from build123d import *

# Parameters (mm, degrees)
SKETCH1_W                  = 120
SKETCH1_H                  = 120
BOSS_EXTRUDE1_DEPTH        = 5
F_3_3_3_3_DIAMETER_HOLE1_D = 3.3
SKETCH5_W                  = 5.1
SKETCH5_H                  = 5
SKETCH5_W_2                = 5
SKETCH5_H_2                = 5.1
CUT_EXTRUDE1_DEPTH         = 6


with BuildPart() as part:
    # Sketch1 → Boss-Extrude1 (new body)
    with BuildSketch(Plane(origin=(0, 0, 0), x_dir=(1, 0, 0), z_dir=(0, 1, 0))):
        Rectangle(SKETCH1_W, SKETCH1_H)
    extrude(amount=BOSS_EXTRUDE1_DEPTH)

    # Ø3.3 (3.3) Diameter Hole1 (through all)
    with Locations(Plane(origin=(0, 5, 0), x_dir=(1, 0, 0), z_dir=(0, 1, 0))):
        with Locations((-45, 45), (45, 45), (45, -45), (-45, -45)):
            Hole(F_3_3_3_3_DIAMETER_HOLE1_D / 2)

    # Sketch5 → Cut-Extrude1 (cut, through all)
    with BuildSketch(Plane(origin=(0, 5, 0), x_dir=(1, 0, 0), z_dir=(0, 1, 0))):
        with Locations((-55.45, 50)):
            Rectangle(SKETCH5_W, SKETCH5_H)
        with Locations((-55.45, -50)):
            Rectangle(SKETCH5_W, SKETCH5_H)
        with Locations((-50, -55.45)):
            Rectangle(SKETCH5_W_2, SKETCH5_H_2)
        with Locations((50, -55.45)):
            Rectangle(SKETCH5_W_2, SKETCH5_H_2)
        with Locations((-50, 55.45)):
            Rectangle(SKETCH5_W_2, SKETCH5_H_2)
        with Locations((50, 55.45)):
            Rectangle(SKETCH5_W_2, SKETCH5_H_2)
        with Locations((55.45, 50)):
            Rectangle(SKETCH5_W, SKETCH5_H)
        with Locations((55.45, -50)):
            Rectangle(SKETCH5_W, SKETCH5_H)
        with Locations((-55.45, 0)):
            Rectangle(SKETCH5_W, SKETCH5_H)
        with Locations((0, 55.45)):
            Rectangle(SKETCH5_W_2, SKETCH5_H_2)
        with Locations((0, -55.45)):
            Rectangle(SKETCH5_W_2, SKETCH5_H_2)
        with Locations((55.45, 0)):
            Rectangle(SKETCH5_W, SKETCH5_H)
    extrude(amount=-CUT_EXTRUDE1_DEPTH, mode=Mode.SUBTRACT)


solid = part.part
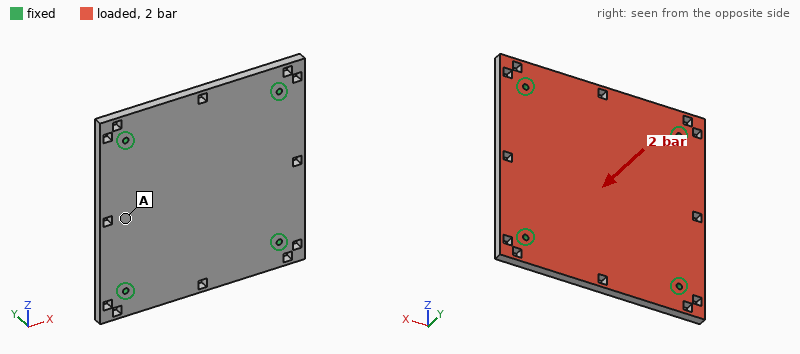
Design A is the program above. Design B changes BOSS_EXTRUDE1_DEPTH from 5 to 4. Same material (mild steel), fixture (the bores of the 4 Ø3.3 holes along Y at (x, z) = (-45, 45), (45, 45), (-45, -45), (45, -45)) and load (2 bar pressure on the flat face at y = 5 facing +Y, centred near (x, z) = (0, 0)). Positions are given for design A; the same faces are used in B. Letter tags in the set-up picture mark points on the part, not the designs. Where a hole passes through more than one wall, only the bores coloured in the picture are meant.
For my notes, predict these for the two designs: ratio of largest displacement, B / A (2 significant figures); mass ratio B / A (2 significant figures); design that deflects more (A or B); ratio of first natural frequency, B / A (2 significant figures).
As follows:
1.9
0.80
B
0.82
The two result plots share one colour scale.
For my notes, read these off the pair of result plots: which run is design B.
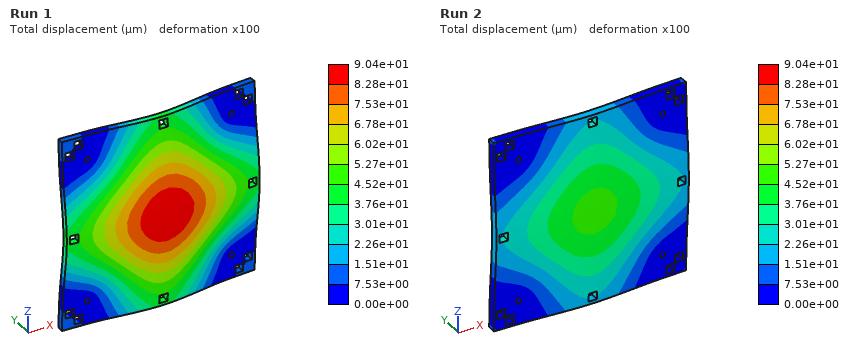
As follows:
Run 1
